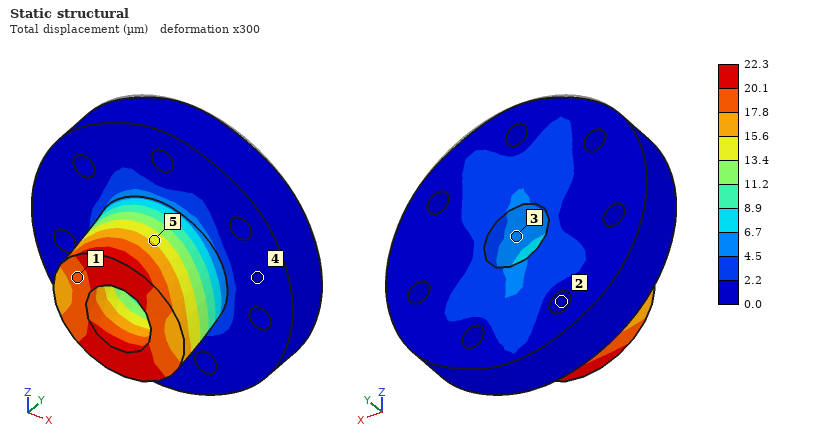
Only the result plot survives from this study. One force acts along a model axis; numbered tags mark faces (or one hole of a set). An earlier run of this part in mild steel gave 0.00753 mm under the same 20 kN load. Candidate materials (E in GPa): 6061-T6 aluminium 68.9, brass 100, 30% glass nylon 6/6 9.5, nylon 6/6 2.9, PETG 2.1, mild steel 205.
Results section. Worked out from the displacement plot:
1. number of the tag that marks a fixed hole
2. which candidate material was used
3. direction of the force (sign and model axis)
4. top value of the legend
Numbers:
2
6061-T6 aluminium
-Z
22.3 µm
